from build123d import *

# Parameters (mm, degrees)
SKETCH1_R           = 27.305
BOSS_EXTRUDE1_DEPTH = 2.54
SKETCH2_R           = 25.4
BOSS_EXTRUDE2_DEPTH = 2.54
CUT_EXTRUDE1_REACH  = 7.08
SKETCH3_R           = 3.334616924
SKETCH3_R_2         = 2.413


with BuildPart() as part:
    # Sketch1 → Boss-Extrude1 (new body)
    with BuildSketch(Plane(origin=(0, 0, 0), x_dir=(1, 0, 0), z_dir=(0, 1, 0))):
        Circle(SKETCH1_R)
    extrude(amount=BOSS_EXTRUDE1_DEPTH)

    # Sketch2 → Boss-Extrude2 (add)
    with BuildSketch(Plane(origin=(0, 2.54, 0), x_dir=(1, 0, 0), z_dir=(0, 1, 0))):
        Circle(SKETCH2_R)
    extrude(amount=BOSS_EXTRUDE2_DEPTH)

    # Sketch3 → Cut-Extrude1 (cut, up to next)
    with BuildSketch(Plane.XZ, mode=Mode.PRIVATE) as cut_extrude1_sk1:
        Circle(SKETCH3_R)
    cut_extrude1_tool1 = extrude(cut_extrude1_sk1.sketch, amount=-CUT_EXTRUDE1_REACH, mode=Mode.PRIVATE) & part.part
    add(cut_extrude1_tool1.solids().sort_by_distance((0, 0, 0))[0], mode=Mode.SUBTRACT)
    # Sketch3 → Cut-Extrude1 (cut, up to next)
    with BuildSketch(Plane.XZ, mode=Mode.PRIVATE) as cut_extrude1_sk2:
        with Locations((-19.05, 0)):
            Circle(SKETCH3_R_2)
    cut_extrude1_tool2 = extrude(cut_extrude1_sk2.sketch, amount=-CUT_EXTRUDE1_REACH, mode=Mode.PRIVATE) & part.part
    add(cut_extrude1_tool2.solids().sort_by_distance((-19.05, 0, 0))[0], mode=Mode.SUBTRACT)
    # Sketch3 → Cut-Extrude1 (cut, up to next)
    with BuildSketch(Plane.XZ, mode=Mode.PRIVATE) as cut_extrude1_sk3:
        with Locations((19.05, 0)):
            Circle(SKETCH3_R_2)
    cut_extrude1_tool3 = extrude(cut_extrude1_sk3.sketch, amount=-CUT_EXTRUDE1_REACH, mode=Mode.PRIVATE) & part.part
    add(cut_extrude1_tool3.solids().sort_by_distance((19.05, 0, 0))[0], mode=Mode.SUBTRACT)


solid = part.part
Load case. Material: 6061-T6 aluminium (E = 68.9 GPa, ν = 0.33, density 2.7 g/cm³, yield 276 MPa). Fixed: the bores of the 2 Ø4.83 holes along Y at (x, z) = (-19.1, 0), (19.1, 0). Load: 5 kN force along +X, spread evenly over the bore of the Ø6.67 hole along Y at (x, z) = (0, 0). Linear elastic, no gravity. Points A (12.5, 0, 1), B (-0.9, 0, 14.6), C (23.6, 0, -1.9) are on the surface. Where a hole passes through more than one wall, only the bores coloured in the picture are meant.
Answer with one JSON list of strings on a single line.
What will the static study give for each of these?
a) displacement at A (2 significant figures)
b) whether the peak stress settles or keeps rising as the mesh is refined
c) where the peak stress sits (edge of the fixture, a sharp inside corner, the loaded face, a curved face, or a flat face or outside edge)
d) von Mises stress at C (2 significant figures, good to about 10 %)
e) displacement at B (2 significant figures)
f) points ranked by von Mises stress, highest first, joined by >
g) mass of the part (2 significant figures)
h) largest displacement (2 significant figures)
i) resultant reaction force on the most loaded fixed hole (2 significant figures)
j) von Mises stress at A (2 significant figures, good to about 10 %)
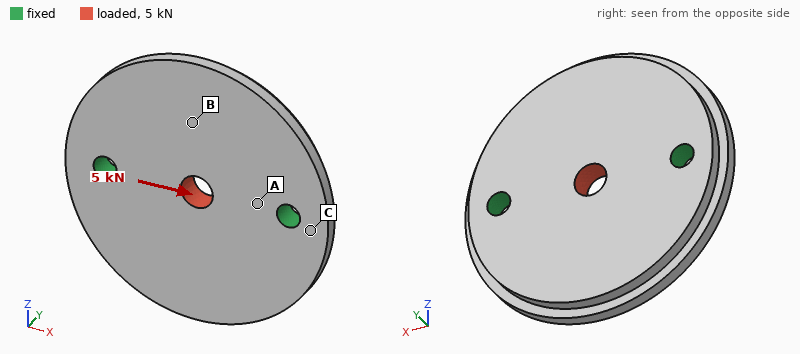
["3.0 µm", "keeps rising", "edge of the fixture", "12 MPa", "4.2 µm", "A > C > B", "29 g", "9.4 µm", "2.5 kN", "45 MPa"]
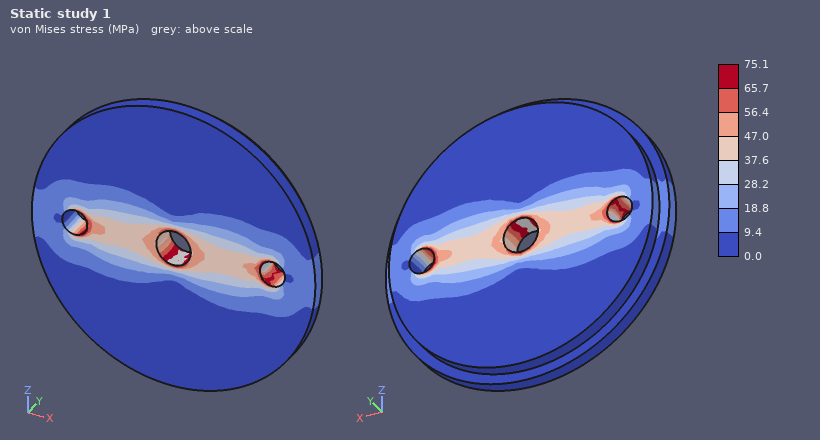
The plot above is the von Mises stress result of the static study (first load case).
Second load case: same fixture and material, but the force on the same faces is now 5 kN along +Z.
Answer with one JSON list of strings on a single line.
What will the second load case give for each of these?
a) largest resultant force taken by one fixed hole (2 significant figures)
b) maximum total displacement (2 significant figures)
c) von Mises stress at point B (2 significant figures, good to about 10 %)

["2.5 kN", "14 µm", "19 MPa"]
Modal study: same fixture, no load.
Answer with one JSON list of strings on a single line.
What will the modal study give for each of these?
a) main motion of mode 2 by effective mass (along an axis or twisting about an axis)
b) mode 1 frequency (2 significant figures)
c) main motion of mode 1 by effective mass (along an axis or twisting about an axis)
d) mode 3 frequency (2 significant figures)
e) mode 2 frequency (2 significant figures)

["along Y", "5700 Hz", "twisting about X", "15 kHz", "7100 Hz"]
